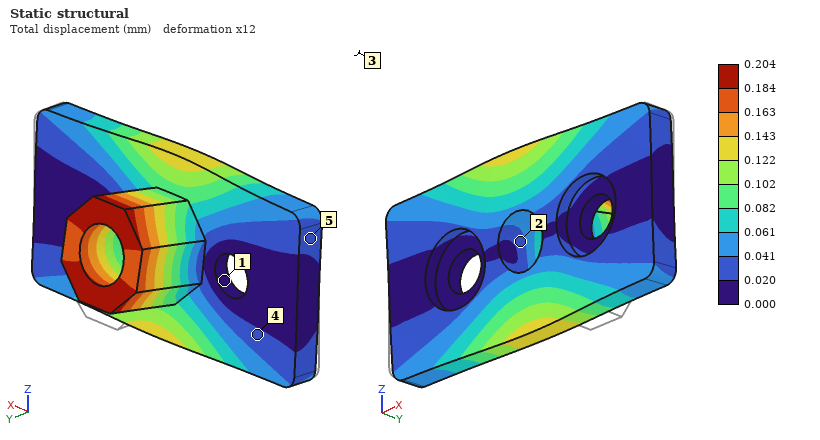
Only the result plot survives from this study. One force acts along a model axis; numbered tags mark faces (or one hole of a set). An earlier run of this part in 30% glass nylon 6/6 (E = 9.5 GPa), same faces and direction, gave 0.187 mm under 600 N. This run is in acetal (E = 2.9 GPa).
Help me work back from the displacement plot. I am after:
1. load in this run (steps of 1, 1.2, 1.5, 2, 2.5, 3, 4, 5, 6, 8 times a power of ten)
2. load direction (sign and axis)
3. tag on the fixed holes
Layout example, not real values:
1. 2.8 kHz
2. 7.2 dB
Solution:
1. 200 N
2. +Z
3. 1
